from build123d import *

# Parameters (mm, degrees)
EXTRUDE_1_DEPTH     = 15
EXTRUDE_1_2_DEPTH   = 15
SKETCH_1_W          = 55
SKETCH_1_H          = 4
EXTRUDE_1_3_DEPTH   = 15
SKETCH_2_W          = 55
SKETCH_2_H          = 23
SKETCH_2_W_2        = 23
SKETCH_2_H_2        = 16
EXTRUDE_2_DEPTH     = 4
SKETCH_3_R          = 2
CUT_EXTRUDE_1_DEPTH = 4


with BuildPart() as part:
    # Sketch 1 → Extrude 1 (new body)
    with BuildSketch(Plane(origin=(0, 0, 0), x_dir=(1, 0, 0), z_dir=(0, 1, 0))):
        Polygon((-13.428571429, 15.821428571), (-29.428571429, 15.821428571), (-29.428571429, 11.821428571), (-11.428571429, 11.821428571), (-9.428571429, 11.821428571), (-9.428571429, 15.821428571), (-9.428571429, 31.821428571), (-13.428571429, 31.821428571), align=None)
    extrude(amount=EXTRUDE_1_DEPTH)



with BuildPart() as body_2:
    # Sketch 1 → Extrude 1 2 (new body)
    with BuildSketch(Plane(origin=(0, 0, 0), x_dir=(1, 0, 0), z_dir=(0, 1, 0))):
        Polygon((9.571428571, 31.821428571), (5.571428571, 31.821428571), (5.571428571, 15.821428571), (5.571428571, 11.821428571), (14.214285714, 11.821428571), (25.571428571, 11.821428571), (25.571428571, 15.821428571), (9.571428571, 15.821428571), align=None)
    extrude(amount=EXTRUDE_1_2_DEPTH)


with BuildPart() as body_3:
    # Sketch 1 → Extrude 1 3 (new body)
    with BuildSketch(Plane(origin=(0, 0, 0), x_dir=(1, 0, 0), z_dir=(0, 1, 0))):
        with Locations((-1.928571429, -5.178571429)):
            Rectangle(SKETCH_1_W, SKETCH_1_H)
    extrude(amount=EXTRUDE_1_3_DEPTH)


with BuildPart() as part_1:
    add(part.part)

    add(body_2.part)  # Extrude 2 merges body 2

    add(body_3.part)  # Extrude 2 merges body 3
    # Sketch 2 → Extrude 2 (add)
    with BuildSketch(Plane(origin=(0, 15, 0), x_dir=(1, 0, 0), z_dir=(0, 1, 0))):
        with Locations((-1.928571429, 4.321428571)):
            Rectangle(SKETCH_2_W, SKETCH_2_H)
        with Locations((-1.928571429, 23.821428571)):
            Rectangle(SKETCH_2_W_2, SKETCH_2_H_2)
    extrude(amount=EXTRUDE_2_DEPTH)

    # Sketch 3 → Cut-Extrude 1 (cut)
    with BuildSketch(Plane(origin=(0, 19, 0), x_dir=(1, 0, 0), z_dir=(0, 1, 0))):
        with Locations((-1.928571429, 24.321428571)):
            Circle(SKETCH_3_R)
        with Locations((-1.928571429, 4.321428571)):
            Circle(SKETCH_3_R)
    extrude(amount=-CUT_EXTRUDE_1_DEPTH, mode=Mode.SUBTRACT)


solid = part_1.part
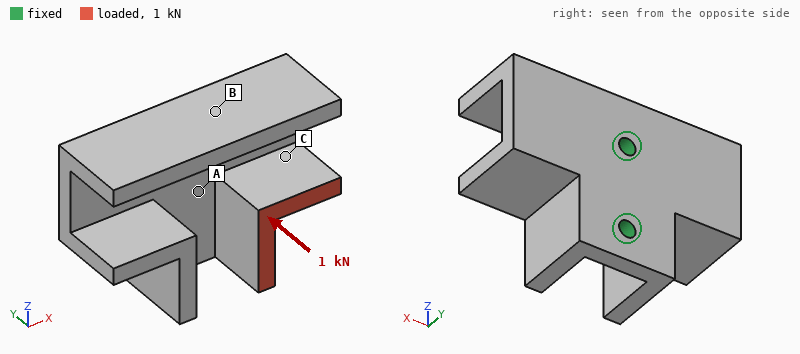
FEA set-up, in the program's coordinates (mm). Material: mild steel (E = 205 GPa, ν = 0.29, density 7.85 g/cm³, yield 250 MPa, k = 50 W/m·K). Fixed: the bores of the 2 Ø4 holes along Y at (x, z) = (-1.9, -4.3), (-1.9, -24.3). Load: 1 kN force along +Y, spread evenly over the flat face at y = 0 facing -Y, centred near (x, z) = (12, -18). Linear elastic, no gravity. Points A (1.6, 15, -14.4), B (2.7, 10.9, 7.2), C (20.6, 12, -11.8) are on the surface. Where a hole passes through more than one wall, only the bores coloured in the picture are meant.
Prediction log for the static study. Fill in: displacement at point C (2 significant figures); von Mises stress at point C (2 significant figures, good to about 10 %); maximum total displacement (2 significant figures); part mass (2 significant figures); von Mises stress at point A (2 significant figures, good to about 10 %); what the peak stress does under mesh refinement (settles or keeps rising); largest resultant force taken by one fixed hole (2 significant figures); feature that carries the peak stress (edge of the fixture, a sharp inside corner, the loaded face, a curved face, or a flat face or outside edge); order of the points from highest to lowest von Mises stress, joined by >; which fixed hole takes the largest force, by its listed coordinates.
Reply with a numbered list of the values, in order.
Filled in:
1. 38 µm
2. 31 MPa
3. 58 µm
4. 110 g
5. 56 MPa
6. keeps rising
7. 670 N
8. edge of the fixture
9. A > C > B
10. (-1.9, -24.3)
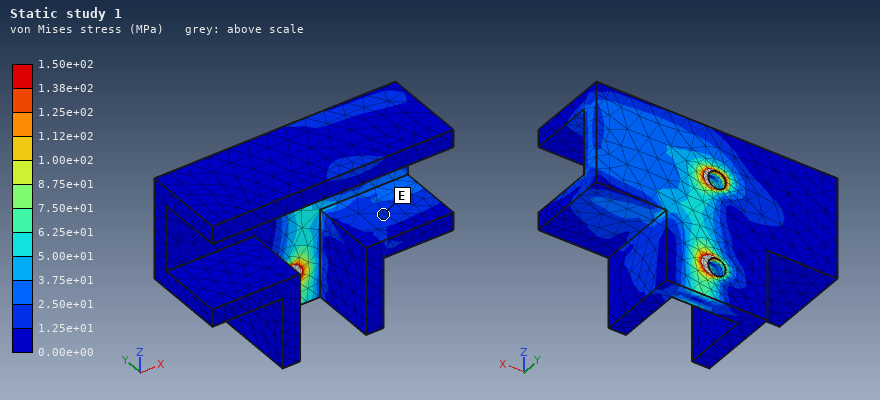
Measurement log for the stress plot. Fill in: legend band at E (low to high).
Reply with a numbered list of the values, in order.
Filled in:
1. 1.25e+01 to 2.50e+01 MPa
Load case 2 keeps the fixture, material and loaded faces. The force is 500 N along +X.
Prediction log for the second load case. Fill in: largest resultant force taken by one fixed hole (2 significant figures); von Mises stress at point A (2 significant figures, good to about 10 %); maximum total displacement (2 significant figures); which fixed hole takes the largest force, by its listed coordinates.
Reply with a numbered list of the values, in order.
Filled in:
1. 360 N
2. 53 MPa
3. 55 µm
4. (-1.9, -24.3)
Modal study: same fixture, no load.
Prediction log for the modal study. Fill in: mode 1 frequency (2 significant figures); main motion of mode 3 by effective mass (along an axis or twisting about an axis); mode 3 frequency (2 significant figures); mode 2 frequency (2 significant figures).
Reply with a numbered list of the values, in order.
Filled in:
1. 3000 Hz
2. along Y
3. 5800 Hz
4. 4800 Hz
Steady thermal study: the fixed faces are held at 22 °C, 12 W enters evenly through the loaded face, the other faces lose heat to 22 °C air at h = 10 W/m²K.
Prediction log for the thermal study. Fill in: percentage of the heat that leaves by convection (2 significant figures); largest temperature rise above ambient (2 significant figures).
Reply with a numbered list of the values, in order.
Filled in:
1. 7.0 %
2. 48 K
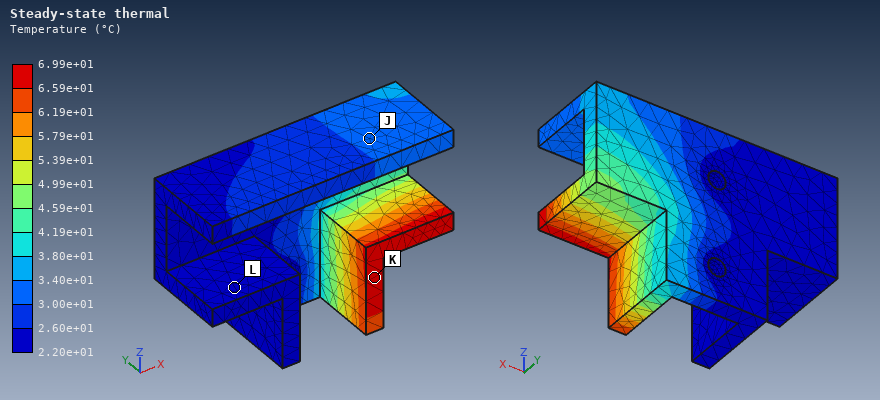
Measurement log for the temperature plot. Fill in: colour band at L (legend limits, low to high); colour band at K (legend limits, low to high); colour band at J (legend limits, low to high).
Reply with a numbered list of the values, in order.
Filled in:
1. 2.20e+01 to 2.60e+01 °C
2. 6.59e+01 to 6.99e+01 °C
3. 3.00e+01 to 3.40e+01 °C
